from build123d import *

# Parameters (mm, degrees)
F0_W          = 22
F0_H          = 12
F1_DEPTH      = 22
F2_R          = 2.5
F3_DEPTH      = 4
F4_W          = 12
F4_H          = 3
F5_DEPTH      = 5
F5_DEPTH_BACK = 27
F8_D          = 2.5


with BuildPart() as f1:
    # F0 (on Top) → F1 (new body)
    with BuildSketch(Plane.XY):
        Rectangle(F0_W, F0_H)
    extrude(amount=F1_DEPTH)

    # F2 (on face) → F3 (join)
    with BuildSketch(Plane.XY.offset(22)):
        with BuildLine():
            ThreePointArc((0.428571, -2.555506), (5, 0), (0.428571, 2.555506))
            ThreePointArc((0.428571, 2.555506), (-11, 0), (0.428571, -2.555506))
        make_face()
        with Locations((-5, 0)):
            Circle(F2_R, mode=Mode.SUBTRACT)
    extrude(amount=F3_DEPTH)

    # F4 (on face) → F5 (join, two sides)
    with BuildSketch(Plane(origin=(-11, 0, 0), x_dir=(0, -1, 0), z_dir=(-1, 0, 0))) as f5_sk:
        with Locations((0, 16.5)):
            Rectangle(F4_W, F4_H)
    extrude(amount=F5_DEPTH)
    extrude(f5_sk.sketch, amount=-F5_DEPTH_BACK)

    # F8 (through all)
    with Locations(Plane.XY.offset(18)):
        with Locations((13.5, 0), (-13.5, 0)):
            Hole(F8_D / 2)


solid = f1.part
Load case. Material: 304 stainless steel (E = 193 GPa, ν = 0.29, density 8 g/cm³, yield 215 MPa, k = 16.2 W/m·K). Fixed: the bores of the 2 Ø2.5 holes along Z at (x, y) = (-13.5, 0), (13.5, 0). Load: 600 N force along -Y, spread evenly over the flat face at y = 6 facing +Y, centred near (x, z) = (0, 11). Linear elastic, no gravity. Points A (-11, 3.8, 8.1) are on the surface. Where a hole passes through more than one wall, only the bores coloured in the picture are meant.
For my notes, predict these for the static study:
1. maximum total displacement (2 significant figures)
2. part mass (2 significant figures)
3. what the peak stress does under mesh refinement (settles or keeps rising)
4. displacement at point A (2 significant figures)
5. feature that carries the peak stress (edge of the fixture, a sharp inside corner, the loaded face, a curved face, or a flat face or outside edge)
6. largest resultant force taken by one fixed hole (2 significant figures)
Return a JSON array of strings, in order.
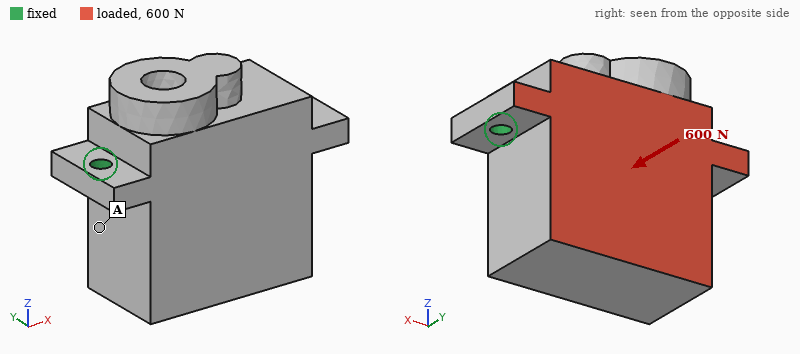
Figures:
["12 µm", "53 g", "keeps rising", "6.7 µm", "edge of the fixture", "300 N"]
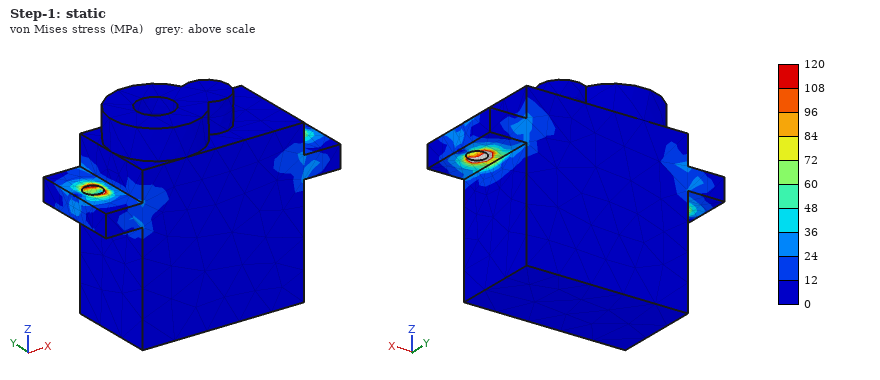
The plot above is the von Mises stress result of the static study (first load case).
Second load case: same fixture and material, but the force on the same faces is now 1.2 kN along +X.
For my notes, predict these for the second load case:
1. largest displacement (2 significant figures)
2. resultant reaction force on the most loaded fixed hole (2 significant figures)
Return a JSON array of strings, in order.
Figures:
["2.9 µm", "710 N"]
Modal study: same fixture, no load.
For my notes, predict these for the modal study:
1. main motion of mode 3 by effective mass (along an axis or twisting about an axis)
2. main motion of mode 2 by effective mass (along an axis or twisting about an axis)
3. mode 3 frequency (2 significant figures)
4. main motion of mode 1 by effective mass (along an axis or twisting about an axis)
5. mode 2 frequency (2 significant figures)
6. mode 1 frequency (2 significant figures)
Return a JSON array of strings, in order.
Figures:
["along X", "along Z", "19 kHz", "along Y", "18 kHz", "5400 Hz"]
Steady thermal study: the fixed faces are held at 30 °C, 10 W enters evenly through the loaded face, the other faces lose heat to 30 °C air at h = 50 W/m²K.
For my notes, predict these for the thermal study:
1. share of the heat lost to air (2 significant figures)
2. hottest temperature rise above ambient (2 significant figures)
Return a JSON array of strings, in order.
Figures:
["28 %", "43 K"]
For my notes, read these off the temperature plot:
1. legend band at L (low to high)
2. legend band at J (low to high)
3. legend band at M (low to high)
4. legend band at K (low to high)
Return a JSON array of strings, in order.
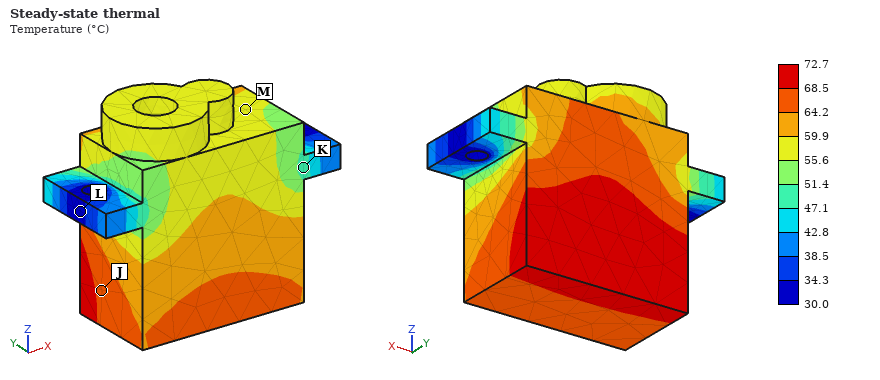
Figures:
["30.0 to 34.3 °C", "64.2 to 68.5 °C", "55.6 to 59.9 °C", "47.1 to 51.4 °C"]
